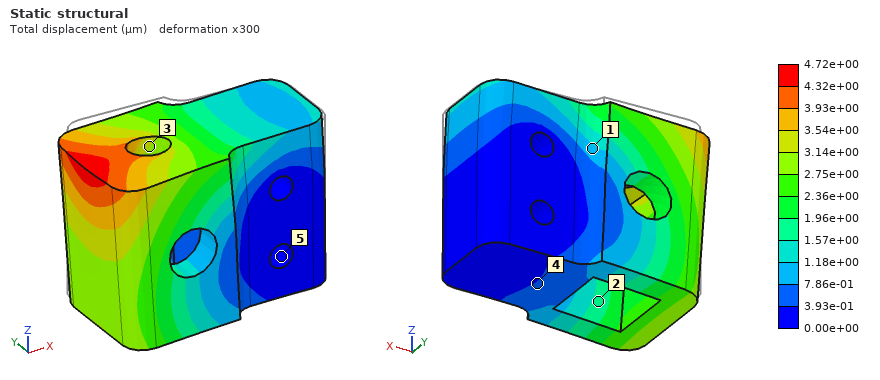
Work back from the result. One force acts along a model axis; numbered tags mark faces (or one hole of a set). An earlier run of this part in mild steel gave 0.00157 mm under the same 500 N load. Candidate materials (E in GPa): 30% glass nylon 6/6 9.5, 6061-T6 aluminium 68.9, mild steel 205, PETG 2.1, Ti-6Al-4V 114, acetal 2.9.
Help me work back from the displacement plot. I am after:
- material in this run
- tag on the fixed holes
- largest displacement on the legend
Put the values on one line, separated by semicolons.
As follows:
6061-T6 aluminium; 5; 4.72e+00 µm
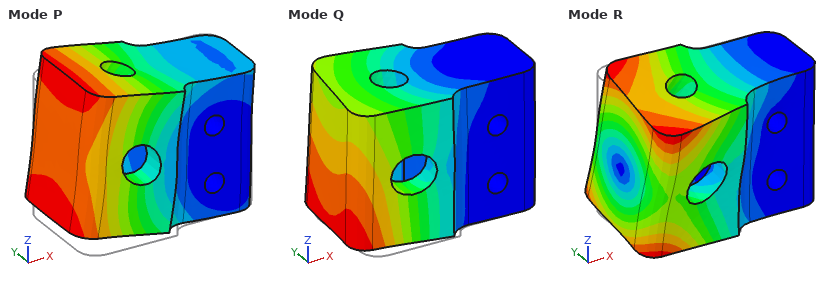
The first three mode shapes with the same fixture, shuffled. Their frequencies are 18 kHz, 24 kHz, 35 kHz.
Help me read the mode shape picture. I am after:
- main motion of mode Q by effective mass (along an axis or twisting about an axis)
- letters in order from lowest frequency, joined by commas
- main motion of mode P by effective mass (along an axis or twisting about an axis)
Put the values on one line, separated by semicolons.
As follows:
along Y; Q, P, R; along Z
